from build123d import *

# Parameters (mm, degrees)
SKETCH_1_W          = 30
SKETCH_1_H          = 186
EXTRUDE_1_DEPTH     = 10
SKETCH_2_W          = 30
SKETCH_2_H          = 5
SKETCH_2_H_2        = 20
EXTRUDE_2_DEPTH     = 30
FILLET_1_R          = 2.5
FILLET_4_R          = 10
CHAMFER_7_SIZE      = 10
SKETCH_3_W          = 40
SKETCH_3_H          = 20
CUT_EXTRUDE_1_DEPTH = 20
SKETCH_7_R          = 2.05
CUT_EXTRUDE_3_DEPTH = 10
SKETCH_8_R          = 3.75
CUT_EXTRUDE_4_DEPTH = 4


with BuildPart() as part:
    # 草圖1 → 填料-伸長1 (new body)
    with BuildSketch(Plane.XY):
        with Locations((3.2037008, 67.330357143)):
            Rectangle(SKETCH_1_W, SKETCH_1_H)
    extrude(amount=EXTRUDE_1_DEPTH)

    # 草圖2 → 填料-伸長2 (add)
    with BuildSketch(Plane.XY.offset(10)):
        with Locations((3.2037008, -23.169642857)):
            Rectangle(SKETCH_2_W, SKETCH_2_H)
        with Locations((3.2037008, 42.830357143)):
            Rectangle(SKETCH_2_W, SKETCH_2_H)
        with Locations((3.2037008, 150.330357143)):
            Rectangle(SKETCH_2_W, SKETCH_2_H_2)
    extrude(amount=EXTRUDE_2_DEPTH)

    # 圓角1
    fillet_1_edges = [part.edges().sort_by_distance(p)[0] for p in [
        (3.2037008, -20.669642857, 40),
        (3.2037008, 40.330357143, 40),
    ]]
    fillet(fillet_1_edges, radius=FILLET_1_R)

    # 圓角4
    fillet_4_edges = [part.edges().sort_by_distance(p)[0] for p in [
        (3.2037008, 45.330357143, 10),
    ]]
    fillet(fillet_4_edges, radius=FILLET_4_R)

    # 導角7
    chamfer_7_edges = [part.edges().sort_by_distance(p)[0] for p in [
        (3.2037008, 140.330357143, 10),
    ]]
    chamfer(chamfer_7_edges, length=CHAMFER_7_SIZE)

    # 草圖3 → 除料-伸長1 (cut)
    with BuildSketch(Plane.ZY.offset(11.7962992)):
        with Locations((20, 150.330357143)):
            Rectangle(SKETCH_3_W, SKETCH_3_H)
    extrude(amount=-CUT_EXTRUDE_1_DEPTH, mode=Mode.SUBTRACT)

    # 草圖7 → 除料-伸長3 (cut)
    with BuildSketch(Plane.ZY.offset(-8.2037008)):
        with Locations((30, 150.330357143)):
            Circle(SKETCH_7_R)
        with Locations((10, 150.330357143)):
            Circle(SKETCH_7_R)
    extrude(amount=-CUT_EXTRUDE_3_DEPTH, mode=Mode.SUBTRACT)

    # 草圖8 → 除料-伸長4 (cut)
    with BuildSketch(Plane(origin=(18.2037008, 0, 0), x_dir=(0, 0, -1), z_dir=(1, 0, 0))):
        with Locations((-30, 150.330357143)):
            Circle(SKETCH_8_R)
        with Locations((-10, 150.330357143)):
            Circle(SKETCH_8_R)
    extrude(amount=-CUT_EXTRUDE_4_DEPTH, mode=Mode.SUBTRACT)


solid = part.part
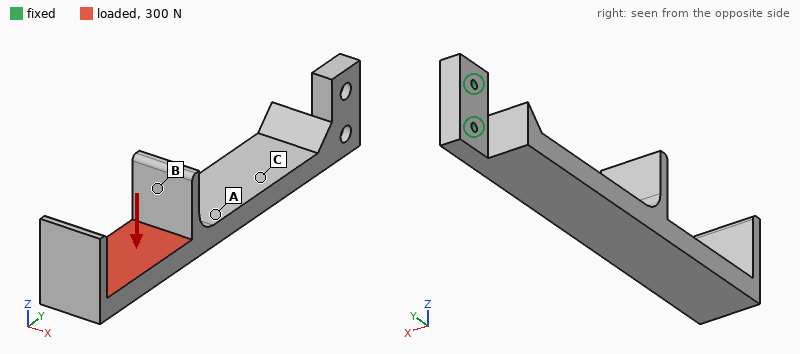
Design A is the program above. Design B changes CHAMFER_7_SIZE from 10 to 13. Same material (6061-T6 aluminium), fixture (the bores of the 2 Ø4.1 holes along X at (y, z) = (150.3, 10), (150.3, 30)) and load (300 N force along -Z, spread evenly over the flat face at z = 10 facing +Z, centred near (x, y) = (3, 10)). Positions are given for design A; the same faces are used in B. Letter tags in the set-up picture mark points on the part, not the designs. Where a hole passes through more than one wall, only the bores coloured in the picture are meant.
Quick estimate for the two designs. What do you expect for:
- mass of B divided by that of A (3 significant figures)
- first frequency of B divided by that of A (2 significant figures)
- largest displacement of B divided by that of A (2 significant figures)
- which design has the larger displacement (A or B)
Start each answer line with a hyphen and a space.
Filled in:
- 1.02
- 1.1
- 0.89
- A
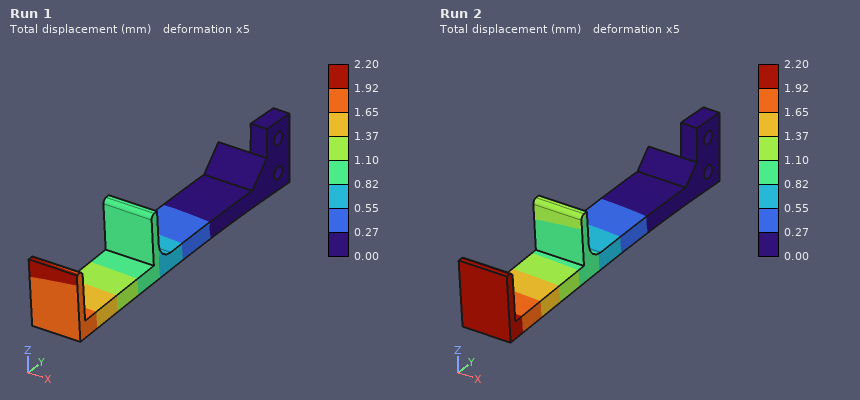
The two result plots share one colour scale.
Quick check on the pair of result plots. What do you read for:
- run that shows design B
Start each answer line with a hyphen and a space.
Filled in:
- Run 1
